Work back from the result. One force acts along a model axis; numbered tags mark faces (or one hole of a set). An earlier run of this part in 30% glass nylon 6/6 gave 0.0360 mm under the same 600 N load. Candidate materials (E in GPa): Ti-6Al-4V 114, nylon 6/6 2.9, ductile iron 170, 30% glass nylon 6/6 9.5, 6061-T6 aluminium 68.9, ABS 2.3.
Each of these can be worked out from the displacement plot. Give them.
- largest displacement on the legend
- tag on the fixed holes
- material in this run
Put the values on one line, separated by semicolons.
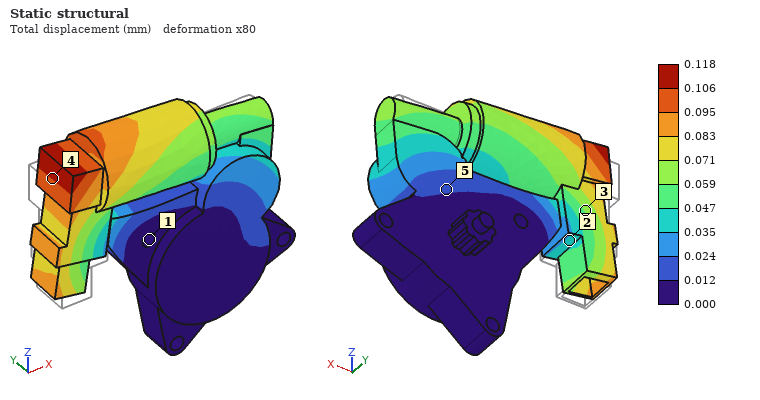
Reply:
0.118 mm; 1; nylon 6/6
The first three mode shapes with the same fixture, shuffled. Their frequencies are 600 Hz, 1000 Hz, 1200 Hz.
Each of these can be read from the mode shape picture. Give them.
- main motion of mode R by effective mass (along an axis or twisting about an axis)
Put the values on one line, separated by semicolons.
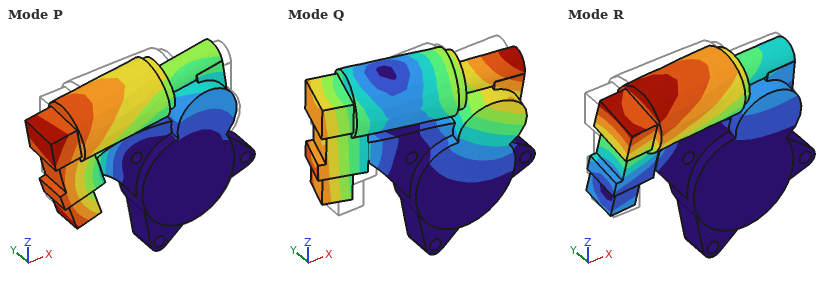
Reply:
along Y
